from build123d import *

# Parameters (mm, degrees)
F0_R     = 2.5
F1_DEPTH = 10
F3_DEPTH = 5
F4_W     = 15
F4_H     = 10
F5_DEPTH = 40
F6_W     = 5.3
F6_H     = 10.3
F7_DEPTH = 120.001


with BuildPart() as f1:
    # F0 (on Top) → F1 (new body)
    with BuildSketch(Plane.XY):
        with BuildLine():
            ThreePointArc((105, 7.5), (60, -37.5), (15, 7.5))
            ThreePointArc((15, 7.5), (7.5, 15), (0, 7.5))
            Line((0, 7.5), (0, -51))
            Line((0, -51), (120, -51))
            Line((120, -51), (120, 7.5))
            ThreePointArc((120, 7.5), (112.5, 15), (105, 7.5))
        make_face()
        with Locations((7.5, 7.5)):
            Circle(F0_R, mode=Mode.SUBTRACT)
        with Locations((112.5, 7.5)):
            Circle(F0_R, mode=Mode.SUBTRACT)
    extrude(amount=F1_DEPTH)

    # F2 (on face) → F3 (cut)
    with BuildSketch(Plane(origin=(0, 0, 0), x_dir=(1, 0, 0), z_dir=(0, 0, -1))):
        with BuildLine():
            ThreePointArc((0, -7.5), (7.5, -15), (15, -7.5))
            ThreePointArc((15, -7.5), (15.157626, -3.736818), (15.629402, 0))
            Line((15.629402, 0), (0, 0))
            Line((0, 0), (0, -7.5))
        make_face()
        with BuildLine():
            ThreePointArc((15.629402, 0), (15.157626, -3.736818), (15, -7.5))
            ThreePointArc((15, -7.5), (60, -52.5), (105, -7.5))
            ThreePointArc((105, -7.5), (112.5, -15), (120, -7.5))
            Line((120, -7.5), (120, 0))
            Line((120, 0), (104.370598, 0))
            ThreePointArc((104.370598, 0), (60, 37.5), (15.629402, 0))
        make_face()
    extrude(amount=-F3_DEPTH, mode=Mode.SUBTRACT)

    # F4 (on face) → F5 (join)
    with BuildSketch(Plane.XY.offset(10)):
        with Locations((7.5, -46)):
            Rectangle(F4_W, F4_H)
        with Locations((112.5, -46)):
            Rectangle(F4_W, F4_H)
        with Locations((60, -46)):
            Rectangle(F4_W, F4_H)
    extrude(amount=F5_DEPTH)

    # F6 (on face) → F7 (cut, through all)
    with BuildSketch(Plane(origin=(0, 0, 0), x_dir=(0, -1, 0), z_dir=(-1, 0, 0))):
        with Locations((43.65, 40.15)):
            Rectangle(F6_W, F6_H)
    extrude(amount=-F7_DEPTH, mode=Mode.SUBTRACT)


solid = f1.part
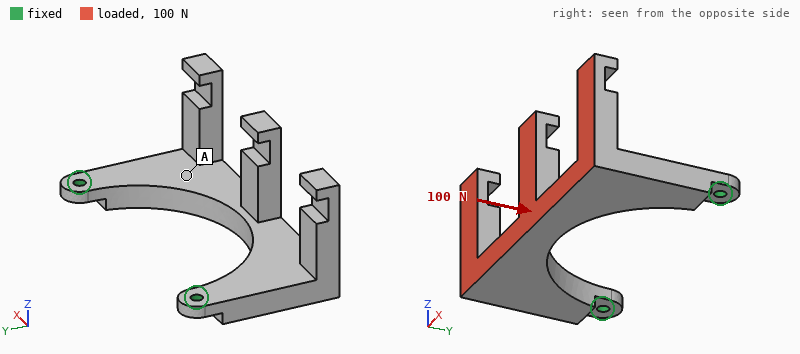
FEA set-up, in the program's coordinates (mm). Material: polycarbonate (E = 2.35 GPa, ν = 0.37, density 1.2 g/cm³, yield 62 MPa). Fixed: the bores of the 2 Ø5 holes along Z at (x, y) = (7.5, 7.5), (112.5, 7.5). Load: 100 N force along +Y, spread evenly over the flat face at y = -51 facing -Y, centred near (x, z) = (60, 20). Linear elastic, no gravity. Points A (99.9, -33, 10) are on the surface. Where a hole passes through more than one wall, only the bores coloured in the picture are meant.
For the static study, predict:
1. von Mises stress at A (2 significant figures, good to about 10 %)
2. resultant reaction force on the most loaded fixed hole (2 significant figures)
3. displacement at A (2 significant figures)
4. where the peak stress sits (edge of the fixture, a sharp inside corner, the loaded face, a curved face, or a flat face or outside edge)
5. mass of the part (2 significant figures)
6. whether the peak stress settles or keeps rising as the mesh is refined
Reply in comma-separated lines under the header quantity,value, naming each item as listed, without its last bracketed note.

quantity,value
von Mises stress at A,1.4 MPa
resultant reaction force on the most loaded fixed hole,53 N
displacement at A,0.59 mm
where the peak stress sits,edge of the fixture
mass of the part,64 g
whether the peak stress settles or keeps rising as the mesh is refined,keeps rising
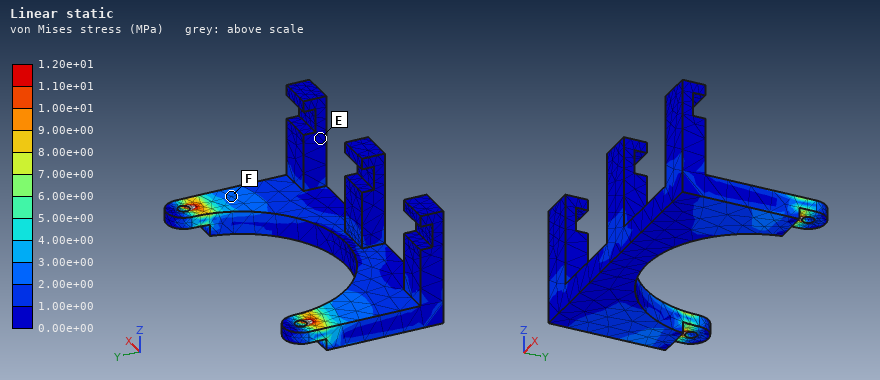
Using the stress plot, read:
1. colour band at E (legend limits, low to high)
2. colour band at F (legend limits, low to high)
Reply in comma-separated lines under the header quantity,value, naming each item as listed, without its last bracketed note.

quantity,value
colour band at E,0.00e+00 to 1.00e+00 MPa
colour band at F,2.00e+00 to 3.00e+00 MPa
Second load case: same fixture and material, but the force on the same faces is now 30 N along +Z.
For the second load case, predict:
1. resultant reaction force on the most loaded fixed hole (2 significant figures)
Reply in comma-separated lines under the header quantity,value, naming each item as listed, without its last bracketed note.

quantity,value
resultant reaction force on the most loaded fixed hole,15 N
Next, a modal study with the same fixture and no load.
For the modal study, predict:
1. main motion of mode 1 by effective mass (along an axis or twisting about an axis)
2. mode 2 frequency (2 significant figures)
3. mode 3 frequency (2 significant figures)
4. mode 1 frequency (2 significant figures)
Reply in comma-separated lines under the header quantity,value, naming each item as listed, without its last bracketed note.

quantity,value
main motion of mode 1 by effective mass,along Z
mode 2 frequency,300 Hz
mode 3 frequency,550 Hz
mode 1 frequency,130 Hz
